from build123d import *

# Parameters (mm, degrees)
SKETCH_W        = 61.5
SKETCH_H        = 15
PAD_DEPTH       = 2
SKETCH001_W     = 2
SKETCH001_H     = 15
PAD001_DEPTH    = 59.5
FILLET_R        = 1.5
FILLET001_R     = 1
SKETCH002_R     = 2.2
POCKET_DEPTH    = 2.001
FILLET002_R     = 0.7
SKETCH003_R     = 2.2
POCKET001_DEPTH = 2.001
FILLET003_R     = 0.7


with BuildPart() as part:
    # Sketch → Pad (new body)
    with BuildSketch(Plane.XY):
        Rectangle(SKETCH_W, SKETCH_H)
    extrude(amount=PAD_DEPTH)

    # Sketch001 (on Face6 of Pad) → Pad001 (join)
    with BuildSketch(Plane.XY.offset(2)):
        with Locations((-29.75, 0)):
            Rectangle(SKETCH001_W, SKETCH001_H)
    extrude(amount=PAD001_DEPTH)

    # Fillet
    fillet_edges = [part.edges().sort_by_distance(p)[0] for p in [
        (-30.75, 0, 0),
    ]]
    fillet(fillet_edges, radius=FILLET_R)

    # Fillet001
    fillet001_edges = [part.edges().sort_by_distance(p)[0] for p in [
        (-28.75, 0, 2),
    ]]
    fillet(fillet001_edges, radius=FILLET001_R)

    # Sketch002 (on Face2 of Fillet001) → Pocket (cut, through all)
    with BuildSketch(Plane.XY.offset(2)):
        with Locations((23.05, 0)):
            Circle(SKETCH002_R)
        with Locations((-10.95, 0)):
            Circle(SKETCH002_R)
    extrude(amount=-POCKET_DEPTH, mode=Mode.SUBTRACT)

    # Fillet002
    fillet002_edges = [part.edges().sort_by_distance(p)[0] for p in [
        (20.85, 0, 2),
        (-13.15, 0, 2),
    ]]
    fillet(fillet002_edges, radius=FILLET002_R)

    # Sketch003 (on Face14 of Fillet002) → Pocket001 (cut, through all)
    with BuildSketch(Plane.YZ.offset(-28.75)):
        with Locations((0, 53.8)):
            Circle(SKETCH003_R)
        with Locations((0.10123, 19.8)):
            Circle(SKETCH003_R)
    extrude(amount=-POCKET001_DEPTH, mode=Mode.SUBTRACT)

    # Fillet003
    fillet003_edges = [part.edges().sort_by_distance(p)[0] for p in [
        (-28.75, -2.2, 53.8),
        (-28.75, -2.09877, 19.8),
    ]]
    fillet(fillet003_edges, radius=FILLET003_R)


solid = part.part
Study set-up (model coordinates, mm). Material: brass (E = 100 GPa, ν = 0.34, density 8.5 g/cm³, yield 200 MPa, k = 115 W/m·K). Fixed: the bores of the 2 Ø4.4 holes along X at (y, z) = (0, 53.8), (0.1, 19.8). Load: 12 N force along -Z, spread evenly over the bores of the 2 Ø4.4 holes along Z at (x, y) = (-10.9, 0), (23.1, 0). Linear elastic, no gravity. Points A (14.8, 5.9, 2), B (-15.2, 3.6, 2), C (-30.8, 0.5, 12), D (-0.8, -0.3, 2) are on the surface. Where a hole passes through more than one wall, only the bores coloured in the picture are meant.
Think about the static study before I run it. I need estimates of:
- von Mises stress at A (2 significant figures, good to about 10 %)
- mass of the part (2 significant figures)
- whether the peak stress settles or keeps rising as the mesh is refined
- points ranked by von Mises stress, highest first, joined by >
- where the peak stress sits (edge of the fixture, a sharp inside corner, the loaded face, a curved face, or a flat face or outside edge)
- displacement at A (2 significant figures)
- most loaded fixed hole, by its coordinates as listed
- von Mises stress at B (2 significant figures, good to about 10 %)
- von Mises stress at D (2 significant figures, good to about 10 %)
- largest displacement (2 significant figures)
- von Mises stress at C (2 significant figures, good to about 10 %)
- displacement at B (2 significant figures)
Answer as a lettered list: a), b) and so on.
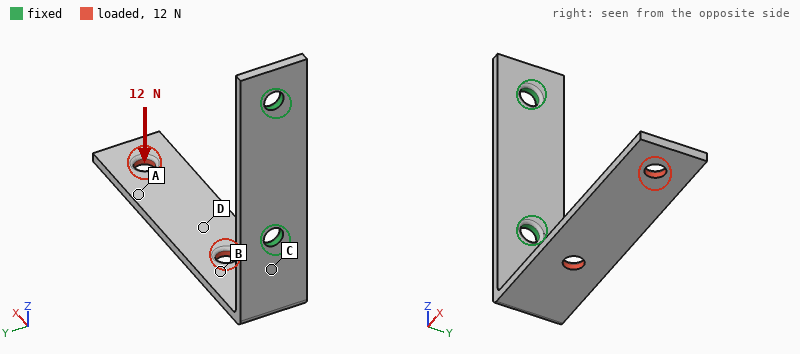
a) 5.1 MPa
b) 30 g
c) keeps rising
d) C > B > D > A
e) edge of the fixture
f) 0.58 mm
g) (0, 53.8)
h) 27 MPa
i) 14 MPa
j) 0.85 mm
k) 38 MPa
l) 0.15 mm
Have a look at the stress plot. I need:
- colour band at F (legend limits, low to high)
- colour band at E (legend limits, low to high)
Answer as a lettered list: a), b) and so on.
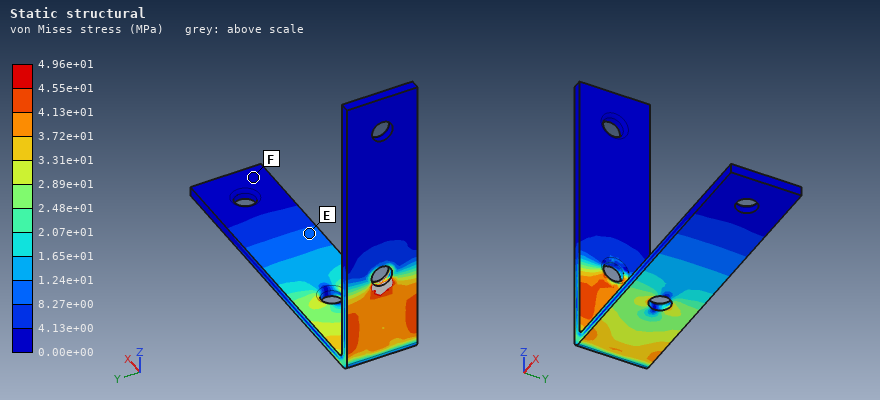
a) 0.00e+00 to 4.13e+00 MPa
b) 8.27e+00 to 1.24e+01 MPa
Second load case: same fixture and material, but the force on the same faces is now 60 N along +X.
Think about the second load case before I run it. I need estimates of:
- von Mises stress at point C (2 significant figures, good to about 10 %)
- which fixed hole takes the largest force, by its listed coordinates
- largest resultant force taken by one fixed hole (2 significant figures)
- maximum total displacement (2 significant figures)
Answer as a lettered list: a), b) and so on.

a) 61 MPa
b) (0.1, 19.8)
c) 63 N
d) 0.65 mm
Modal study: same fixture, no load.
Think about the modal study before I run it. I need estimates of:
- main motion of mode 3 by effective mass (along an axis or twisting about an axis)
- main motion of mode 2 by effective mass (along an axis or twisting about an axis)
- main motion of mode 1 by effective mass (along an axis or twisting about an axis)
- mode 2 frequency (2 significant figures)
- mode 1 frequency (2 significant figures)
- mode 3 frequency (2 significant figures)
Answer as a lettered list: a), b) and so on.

a) along X
b) along Y
c) along Z
d) 350 Hz
e) 210 Hz
f) 1100 Hz
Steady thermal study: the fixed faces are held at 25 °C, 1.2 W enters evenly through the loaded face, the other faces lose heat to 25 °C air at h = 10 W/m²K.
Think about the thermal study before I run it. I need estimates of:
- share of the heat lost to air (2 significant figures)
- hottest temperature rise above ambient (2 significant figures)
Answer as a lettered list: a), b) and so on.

a) 21 %
b) 16 K
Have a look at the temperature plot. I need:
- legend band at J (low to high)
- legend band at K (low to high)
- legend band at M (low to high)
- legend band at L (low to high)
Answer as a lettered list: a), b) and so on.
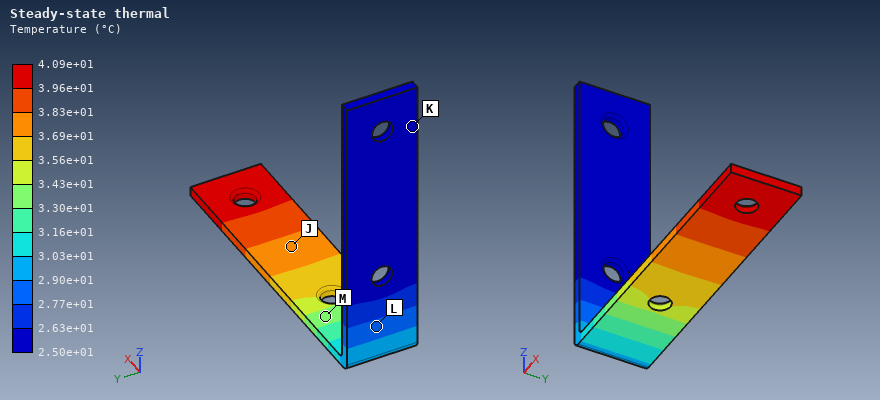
a) 3.69e+01 to 3.83e+01 °C
b) 2.50e+01 to 2.63e+01 °C
c) 3.30e+01 to 3.43e+01 °C
d) 2.77e+01 to 2.90e+01 °C
